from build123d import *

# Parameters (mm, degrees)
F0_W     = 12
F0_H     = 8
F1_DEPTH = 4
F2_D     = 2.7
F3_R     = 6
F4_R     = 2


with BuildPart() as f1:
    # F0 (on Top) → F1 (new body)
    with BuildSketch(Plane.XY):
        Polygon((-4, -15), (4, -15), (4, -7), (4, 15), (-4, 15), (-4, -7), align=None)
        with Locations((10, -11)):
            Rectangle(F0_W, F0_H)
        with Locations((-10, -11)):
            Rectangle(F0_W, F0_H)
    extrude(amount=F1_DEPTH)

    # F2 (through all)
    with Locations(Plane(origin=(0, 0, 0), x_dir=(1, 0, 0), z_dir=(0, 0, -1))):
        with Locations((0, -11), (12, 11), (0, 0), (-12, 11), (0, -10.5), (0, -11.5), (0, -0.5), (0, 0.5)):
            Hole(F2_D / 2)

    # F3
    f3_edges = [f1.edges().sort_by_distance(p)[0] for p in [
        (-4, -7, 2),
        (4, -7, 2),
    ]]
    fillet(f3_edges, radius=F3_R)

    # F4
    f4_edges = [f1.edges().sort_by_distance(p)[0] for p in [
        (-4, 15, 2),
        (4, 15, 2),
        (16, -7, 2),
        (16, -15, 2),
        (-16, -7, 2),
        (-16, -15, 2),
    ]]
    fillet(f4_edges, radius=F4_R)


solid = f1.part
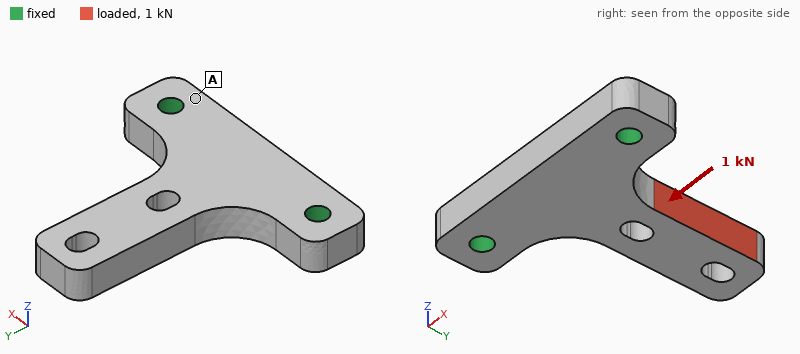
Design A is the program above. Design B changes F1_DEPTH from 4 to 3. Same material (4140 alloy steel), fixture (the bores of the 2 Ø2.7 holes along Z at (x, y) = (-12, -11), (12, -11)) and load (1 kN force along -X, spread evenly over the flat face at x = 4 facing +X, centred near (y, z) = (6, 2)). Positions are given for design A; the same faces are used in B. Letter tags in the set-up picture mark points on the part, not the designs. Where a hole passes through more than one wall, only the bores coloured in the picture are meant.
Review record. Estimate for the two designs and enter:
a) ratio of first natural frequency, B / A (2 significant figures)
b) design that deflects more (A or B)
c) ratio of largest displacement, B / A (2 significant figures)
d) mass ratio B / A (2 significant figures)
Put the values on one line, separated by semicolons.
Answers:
0.78; B; 1.3; 0.75
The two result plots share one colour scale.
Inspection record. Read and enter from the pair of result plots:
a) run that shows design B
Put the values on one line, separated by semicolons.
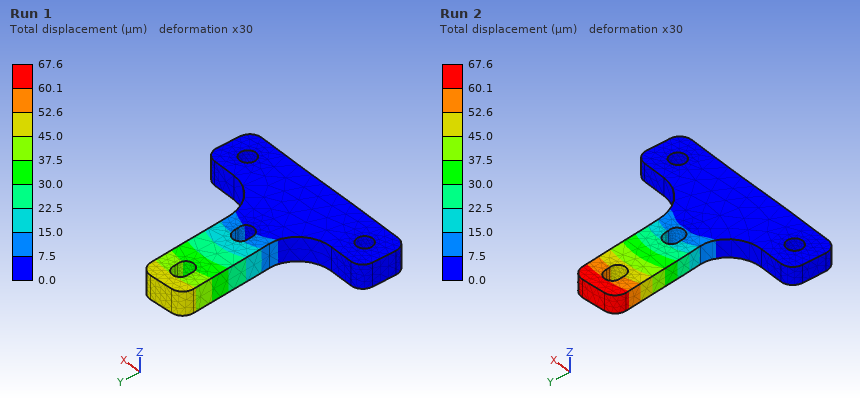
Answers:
Run 2
